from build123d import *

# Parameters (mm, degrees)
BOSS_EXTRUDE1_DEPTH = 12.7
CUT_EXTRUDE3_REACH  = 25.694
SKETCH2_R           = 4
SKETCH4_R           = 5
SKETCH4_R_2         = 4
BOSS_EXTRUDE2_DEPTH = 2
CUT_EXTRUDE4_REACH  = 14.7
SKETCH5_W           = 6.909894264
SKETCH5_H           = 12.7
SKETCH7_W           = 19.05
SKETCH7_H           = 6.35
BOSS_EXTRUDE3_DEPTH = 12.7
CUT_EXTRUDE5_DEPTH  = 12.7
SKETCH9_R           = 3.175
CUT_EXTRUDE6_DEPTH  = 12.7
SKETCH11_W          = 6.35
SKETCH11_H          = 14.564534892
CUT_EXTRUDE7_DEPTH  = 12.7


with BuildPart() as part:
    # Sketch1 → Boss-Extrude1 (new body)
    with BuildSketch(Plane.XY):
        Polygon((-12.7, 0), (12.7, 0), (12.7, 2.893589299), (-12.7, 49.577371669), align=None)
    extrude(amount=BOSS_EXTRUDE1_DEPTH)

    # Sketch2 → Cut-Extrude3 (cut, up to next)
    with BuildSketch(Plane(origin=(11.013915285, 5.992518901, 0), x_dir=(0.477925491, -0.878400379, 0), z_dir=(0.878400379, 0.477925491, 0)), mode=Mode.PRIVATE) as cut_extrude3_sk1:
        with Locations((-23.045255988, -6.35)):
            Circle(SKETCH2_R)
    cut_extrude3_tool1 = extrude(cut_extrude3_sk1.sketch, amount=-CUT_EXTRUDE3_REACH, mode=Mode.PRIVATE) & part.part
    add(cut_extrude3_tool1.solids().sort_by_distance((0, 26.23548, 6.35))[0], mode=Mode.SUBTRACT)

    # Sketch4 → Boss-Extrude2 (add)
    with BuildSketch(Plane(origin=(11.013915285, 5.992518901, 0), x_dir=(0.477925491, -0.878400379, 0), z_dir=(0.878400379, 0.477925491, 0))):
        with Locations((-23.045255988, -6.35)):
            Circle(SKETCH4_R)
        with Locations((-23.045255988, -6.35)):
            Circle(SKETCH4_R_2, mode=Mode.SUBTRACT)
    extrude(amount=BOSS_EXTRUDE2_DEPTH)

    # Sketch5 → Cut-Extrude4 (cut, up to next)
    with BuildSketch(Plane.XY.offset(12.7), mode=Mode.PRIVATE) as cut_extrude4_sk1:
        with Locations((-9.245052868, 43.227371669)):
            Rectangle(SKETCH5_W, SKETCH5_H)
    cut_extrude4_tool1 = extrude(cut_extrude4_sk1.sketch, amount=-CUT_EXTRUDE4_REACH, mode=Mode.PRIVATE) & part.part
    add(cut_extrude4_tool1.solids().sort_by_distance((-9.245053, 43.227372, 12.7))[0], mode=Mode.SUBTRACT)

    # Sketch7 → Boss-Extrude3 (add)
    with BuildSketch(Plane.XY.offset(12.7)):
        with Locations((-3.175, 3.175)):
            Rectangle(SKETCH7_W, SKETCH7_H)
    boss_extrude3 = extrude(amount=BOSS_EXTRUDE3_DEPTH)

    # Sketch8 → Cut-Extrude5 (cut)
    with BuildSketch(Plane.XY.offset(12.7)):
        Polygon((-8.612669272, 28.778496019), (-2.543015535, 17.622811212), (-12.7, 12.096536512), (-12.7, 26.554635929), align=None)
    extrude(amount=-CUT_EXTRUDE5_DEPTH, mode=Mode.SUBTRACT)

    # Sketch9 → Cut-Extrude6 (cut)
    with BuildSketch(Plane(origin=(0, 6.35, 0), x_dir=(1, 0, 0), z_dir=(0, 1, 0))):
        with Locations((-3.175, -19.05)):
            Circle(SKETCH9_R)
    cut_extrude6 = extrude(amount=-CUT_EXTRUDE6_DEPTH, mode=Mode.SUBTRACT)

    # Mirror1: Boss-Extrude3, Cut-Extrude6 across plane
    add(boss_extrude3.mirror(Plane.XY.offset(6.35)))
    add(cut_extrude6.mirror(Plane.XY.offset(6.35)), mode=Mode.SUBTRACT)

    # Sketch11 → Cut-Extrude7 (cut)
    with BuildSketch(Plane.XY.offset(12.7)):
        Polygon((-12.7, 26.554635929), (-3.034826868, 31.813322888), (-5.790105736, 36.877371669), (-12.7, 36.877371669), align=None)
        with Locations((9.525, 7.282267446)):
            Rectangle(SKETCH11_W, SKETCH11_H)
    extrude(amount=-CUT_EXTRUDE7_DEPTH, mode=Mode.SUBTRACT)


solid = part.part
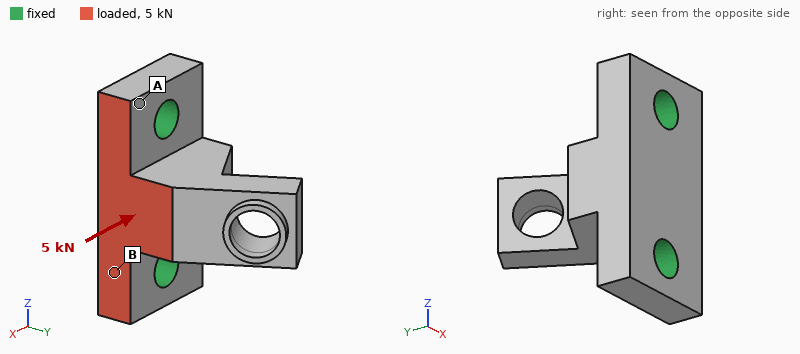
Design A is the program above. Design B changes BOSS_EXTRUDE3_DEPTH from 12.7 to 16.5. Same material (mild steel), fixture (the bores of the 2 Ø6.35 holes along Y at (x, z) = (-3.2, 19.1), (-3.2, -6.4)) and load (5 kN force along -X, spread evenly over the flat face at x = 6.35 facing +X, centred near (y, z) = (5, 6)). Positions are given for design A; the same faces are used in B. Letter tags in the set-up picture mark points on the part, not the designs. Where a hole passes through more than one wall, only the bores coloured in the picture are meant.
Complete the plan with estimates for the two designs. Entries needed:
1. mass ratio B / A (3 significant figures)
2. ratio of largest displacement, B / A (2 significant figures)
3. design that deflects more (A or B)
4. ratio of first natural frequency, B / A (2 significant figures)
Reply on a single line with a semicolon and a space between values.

1.12; 0.85; A; 1.0
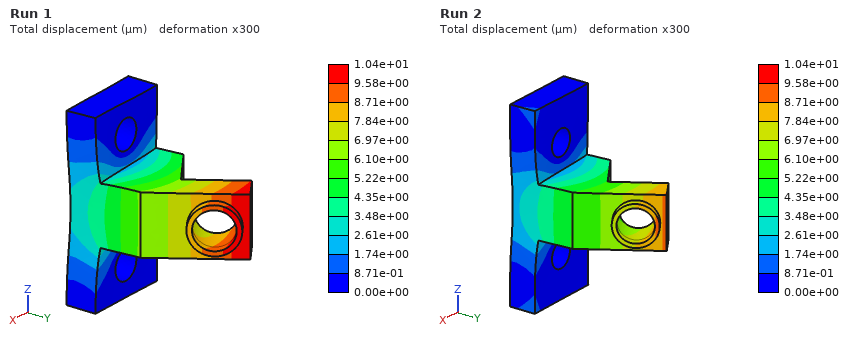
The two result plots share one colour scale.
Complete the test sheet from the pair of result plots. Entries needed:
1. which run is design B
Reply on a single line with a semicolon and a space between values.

Run 2
